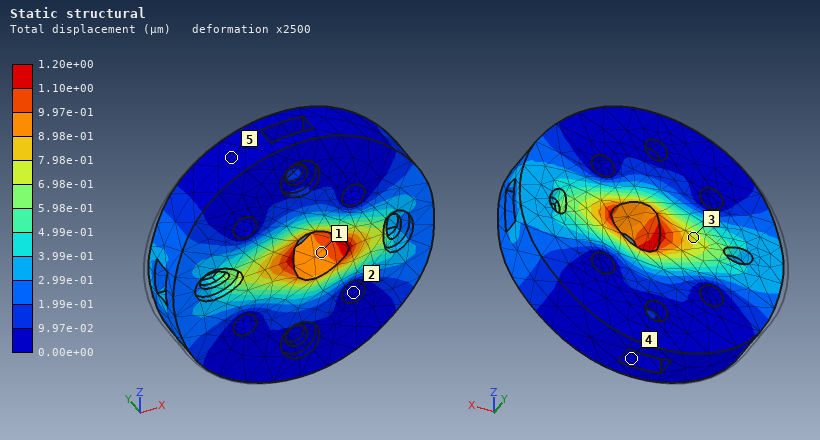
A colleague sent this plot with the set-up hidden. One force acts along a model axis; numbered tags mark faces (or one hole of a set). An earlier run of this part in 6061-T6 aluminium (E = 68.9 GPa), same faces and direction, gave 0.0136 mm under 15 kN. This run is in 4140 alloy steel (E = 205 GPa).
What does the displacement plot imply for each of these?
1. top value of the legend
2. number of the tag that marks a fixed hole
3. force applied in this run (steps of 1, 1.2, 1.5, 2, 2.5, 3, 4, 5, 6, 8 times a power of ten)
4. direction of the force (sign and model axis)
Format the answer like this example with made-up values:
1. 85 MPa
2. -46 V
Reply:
1. 1.20e+00 µm
2. 2
3. 4 kN
4. +X
